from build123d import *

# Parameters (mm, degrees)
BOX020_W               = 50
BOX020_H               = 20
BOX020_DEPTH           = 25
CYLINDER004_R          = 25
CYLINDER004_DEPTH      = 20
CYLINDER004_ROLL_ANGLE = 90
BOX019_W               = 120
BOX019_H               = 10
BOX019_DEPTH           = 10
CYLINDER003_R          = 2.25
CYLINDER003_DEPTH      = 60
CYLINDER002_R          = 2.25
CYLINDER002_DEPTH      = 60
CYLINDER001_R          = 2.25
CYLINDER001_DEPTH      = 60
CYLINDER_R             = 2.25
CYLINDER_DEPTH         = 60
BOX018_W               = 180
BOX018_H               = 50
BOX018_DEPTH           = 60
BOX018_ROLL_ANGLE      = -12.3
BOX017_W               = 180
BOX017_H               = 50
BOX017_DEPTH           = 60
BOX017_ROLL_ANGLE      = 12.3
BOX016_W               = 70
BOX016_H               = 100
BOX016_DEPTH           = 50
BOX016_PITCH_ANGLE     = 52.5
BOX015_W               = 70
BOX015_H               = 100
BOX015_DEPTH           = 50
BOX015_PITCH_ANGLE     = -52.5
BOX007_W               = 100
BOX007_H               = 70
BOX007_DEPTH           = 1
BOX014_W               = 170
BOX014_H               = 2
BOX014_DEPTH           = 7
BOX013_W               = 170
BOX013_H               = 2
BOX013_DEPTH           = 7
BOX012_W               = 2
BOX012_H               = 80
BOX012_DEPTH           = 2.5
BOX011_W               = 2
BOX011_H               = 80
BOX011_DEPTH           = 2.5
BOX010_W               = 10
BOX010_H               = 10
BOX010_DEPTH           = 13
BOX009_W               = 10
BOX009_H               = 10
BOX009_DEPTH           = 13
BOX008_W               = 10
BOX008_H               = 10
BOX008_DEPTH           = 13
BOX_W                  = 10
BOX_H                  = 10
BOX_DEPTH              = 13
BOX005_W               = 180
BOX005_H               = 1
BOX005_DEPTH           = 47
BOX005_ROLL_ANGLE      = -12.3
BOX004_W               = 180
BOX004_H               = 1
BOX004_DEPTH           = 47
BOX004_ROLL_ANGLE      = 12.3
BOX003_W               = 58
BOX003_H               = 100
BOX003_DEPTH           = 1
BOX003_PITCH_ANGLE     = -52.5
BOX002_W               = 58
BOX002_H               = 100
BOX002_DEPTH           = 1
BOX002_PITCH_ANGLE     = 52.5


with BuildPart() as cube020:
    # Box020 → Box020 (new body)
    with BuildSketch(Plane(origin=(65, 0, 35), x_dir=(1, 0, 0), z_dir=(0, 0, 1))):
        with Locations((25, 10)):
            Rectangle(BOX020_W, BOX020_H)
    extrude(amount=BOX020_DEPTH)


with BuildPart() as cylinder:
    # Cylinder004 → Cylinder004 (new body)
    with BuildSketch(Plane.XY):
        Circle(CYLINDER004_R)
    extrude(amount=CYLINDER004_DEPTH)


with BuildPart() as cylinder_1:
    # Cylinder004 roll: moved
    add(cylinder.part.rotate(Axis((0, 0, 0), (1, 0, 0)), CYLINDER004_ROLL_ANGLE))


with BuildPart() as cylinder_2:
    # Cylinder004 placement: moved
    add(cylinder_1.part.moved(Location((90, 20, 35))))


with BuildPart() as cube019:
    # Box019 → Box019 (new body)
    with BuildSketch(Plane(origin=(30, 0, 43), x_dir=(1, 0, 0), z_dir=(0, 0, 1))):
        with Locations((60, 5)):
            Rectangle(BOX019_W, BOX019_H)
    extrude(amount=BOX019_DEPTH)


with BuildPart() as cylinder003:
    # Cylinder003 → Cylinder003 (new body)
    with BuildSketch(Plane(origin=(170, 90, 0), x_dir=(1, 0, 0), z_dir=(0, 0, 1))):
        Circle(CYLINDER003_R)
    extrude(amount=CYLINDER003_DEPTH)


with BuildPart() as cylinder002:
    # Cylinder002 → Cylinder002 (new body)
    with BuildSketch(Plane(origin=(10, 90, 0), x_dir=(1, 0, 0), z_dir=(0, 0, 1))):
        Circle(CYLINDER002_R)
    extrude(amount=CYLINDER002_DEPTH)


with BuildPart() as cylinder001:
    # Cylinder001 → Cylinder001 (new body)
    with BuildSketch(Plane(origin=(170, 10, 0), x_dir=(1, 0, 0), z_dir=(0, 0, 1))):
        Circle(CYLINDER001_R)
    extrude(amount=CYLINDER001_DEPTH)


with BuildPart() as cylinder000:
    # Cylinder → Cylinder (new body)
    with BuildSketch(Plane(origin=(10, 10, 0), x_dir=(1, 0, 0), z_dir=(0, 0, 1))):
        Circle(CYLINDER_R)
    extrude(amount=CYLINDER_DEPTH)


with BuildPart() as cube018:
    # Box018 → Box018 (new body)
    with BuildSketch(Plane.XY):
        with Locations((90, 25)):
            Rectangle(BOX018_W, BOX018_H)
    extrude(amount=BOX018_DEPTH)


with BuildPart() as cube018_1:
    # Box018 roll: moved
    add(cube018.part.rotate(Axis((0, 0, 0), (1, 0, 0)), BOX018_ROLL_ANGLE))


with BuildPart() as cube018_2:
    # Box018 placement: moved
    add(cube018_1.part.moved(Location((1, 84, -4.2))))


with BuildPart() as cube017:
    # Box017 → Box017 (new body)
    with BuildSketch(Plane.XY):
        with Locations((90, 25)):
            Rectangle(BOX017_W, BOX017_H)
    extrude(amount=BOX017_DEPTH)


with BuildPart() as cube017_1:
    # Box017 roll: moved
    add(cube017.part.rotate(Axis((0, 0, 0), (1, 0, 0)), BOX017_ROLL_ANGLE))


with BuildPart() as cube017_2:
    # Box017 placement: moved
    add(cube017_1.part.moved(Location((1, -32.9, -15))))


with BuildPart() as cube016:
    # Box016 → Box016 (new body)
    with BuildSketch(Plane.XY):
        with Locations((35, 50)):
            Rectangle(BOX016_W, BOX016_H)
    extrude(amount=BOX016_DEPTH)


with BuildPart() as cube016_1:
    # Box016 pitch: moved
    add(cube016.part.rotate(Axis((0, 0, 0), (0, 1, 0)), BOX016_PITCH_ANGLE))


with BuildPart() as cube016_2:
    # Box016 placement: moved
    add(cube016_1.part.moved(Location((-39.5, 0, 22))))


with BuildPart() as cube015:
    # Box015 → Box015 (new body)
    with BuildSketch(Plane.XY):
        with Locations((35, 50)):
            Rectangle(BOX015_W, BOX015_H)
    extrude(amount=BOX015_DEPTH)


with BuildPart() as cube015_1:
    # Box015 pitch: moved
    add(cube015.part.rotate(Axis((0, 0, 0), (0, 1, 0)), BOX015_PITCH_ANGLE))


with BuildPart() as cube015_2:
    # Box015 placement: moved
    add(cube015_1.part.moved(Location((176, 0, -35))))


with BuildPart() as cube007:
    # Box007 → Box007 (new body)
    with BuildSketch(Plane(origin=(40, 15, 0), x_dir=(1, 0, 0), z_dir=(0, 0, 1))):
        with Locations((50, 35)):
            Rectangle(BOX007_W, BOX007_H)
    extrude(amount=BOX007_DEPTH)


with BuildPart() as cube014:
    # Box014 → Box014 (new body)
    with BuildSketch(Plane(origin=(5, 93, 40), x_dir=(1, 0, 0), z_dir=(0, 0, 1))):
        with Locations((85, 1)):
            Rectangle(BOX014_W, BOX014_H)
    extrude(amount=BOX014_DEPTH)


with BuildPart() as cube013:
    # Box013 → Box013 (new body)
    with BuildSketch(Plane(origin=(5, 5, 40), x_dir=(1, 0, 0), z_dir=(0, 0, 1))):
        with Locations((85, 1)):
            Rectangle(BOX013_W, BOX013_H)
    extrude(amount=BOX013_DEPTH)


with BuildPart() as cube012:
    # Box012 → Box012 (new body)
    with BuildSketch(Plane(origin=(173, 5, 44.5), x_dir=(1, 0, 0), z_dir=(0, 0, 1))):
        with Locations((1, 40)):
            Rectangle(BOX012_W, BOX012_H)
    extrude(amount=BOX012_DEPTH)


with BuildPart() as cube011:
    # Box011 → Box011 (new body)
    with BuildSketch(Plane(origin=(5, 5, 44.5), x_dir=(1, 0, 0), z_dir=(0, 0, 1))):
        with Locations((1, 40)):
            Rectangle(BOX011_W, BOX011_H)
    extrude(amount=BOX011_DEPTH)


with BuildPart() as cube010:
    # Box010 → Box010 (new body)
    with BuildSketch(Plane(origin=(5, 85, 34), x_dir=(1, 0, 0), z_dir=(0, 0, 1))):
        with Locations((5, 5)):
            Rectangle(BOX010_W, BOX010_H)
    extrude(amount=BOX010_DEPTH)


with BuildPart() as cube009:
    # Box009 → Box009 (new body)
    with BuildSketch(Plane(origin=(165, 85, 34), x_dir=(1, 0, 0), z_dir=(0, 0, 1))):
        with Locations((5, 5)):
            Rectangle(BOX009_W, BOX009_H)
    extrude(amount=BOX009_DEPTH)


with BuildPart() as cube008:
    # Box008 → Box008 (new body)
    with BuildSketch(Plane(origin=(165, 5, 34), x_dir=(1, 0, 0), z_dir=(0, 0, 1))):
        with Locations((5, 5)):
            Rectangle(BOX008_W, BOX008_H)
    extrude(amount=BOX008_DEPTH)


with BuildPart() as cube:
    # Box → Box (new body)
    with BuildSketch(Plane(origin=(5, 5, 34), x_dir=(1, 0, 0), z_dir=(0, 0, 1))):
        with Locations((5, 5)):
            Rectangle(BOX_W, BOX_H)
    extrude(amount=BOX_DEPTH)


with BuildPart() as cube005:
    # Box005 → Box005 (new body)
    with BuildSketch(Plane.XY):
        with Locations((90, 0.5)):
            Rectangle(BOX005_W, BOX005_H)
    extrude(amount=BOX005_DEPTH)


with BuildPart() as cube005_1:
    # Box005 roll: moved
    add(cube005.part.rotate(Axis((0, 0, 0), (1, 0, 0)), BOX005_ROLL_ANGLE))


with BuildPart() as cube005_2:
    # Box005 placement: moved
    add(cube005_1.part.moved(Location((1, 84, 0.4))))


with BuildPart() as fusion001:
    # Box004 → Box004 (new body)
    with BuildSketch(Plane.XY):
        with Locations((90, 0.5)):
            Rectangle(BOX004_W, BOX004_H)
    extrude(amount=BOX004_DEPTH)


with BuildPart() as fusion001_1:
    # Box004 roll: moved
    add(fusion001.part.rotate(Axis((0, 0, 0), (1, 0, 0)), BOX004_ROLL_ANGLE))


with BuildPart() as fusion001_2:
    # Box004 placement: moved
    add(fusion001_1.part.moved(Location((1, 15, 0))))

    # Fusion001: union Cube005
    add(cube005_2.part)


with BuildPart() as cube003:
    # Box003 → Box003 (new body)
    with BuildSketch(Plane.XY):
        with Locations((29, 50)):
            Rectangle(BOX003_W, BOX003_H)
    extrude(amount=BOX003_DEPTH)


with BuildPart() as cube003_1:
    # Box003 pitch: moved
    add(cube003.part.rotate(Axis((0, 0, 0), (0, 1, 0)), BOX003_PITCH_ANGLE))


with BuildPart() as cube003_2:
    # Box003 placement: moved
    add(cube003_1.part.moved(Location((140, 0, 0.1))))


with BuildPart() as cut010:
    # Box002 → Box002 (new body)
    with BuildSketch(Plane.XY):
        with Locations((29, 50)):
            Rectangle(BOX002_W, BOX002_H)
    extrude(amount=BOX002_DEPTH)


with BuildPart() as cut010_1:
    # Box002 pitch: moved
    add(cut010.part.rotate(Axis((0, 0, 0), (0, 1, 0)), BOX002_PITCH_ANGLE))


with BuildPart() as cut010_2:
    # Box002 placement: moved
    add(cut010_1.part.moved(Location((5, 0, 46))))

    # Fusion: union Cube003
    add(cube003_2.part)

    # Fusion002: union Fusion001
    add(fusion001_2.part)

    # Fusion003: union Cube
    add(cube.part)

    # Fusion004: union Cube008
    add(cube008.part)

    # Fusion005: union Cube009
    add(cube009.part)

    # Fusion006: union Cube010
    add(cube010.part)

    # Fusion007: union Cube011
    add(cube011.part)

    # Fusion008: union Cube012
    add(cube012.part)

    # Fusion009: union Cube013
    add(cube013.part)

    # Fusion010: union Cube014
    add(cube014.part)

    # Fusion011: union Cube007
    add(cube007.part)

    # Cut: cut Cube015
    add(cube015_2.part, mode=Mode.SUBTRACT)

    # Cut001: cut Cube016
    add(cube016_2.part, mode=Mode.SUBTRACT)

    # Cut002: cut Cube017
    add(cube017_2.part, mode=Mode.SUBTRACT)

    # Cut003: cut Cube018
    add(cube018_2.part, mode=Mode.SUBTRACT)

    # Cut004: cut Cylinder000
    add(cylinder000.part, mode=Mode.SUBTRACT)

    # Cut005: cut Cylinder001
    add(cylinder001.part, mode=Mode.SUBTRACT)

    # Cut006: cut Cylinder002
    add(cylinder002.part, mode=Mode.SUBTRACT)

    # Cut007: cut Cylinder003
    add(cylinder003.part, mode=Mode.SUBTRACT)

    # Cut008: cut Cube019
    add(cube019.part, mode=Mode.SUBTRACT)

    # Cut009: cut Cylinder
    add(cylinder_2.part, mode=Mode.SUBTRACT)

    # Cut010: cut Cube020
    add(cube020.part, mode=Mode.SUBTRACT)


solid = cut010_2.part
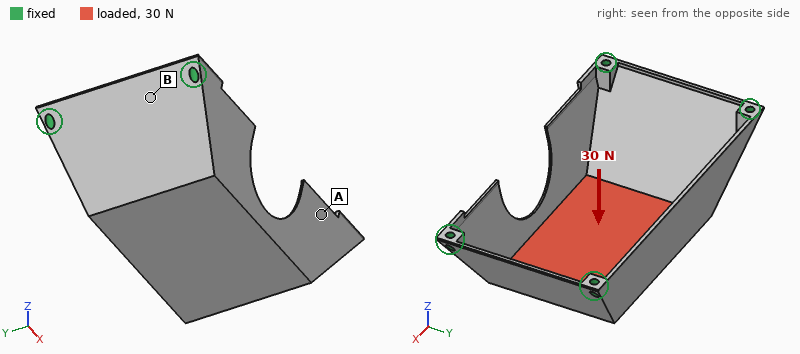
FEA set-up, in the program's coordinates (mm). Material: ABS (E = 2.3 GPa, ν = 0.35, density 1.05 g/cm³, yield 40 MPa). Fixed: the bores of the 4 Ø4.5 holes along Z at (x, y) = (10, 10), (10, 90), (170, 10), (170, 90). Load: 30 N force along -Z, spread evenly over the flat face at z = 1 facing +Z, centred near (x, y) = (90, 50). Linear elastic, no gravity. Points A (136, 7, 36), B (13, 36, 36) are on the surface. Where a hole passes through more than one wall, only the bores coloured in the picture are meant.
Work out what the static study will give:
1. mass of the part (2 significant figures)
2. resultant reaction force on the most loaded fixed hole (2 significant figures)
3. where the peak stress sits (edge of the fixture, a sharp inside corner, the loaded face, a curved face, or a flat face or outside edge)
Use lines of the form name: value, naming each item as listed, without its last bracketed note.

mass of the part: 30 g
resultant reaction force on the most loaded fixed hole: 12 N
where the peak stress sits: a flat face or outside edge
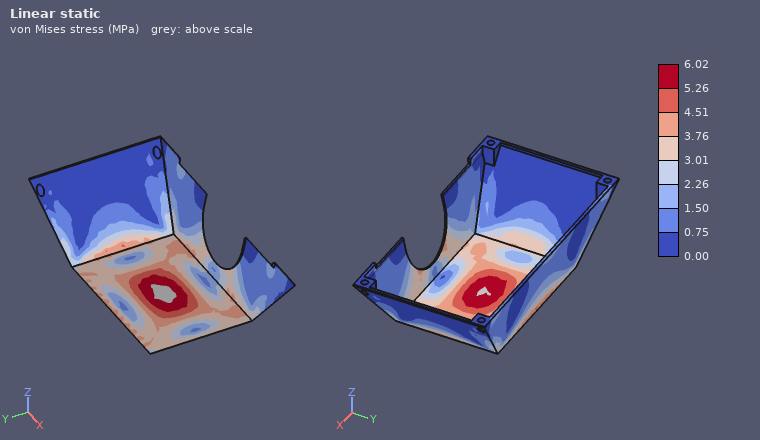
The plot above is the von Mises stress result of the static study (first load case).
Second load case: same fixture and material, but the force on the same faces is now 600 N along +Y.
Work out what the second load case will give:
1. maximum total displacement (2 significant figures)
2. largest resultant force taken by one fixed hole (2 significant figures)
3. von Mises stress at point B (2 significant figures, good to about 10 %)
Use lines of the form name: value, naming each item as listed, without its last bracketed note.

maximum total displacement: 0.55 mm
largest resultant force taken by one fixed hole: 230 N
von Mises stress at point B: 3.9 MPa
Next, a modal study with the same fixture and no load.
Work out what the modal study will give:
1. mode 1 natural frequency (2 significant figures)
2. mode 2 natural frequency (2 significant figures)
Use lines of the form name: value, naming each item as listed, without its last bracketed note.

mode 1 natural frequency: 150 Hz
mode 2 natural frequency: 240 Hz
